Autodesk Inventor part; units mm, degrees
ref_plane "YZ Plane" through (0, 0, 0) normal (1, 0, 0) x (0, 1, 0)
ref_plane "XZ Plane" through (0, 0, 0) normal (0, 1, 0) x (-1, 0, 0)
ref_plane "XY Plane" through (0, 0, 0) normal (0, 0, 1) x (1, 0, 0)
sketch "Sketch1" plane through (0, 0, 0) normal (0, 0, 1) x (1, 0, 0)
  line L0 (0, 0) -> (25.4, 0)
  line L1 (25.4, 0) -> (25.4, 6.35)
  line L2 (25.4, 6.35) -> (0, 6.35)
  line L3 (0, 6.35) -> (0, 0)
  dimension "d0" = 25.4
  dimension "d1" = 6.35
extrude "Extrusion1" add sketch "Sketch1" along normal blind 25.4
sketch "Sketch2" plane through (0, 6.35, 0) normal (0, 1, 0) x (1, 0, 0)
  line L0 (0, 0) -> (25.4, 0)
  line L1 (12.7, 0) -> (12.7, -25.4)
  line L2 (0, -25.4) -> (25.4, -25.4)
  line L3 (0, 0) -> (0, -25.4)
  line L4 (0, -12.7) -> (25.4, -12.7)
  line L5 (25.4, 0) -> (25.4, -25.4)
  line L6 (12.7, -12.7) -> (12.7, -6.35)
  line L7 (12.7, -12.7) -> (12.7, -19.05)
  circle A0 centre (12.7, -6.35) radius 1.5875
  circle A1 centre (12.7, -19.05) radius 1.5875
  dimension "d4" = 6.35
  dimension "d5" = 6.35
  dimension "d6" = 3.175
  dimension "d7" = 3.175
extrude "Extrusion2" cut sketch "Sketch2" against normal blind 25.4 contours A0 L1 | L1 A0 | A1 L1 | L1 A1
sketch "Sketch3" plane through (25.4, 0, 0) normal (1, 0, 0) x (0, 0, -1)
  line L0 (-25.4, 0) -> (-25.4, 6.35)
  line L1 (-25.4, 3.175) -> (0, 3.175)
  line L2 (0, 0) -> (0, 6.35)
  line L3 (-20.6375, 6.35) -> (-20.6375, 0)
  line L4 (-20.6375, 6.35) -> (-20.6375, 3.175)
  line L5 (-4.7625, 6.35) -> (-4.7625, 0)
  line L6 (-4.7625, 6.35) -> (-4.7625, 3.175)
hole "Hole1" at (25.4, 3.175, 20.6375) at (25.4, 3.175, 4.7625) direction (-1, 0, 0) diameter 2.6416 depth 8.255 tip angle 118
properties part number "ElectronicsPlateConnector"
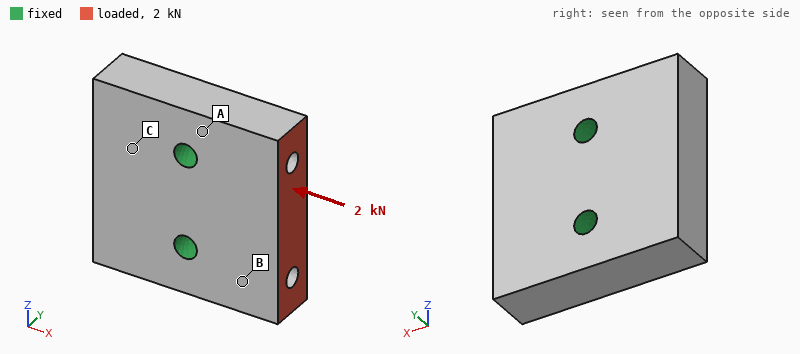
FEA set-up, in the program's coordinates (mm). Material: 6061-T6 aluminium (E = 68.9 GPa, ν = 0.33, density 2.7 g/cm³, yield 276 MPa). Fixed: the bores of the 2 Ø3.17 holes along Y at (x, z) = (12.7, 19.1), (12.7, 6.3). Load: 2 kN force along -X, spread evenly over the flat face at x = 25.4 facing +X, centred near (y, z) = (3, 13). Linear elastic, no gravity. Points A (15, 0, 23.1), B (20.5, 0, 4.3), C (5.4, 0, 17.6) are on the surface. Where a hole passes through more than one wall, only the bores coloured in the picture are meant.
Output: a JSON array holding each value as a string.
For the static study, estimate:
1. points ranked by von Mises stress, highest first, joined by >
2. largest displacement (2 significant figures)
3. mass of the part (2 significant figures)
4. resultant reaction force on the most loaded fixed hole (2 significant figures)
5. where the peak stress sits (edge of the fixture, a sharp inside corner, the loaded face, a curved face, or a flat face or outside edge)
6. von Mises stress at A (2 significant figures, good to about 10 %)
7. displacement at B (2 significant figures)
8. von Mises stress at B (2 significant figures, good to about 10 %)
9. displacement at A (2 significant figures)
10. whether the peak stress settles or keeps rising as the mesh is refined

["B > A > C", "3.2 µm", "11 g", "1.0 kN", "edge of the fixture", "9.1 MPa", "1.9 µm", "15 MPa", "1.1 µm", "keeps rising"]
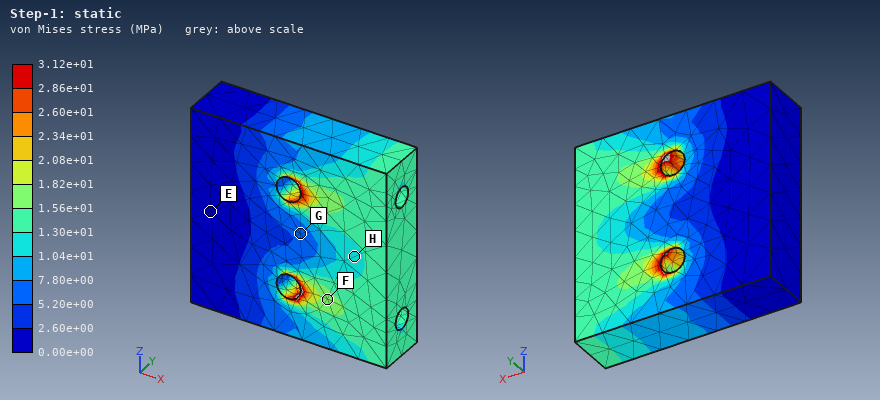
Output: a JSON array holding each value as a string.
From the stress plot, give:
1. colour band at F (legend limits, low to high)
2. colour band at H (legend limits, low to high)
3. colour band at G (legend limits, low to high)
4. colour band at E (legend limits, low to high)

["1.56e+01 to 1.82e+01 MPa", "1.04e+01 to 1.30e+01 MPa", "5.20e+00 to 7.80e+00 MPa", "0.00e+00 to 2.60e+00 MPa"]
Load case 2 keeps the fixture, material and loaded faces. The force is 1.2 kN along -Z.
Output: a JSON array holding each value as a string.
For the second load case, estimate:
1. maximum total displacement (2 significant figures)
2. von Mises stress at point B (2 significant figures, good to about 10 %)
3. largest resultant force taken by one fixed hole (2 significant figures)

["10.0 µm", "13 MPa", "1.2 kN"]
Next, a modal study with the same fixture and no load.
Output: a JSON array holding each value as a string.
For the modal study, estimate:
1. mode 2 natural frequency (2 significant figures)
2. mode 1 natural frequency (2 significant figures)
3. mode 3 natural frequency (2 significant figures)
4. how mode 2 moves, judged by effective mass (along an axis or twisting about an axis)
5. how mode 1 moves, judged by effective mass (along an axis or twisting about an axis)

["30 kHz", "25 kHz", "35 kHz", "along Y", "twisting about Z"]
